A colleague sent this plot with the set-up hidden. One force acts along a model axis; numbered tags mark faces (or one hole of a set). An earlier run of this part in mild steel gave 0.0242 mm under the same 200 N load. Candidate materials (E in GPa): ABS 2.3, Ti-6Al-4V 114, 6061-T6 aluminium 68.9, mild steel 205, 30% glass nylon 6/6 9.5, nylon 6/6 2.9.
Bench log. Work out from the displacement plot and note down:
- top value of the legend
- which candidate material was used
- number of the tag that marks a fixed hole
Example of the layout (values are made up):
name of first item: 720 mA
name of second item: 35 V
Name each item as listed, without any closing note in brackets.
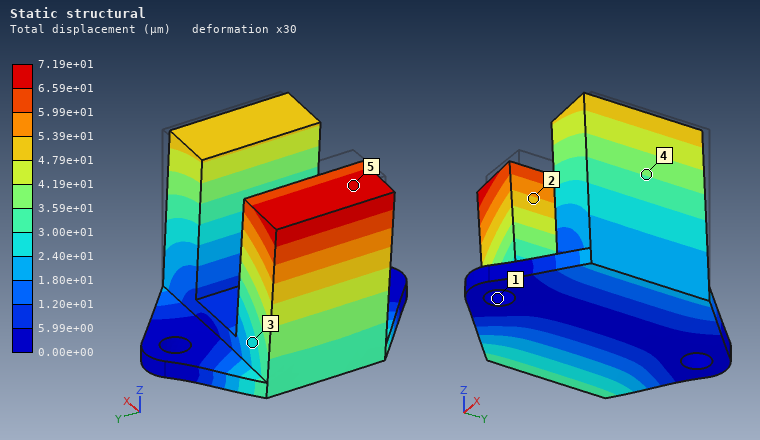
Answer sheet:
top value of the legend: 7.19e+01 µm
which candidate material was used: 6061-T6 aluminium
number of the tag that marks a fixed hole: 1
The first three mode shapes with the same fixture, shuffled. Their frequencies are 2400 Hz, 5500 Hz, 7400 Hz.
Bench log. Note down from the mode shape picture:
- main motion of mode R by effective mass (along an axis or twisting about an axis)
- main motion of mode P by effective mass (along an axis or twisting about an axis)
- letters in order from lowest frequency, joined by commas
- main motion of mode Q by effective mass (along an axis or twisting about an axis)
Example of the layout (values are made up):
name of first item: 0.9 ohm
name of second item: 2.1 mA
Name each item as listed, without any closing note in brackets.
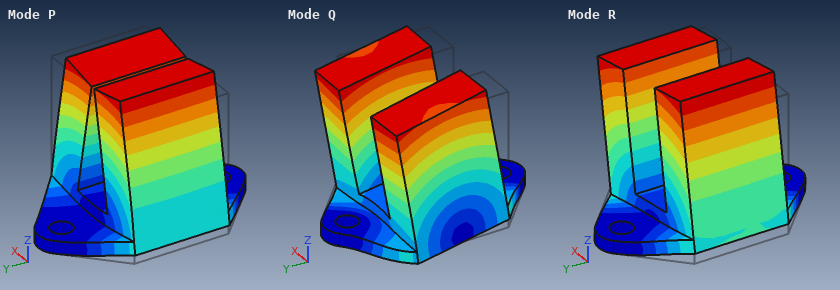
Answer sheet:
main motion of mode R by effective mass: along X
main motion of mode P by effective mass: along Z
letters in order from lowest frequency, joined by commas: R, P, Q
main motion of mode Q by effective mass: along Y
